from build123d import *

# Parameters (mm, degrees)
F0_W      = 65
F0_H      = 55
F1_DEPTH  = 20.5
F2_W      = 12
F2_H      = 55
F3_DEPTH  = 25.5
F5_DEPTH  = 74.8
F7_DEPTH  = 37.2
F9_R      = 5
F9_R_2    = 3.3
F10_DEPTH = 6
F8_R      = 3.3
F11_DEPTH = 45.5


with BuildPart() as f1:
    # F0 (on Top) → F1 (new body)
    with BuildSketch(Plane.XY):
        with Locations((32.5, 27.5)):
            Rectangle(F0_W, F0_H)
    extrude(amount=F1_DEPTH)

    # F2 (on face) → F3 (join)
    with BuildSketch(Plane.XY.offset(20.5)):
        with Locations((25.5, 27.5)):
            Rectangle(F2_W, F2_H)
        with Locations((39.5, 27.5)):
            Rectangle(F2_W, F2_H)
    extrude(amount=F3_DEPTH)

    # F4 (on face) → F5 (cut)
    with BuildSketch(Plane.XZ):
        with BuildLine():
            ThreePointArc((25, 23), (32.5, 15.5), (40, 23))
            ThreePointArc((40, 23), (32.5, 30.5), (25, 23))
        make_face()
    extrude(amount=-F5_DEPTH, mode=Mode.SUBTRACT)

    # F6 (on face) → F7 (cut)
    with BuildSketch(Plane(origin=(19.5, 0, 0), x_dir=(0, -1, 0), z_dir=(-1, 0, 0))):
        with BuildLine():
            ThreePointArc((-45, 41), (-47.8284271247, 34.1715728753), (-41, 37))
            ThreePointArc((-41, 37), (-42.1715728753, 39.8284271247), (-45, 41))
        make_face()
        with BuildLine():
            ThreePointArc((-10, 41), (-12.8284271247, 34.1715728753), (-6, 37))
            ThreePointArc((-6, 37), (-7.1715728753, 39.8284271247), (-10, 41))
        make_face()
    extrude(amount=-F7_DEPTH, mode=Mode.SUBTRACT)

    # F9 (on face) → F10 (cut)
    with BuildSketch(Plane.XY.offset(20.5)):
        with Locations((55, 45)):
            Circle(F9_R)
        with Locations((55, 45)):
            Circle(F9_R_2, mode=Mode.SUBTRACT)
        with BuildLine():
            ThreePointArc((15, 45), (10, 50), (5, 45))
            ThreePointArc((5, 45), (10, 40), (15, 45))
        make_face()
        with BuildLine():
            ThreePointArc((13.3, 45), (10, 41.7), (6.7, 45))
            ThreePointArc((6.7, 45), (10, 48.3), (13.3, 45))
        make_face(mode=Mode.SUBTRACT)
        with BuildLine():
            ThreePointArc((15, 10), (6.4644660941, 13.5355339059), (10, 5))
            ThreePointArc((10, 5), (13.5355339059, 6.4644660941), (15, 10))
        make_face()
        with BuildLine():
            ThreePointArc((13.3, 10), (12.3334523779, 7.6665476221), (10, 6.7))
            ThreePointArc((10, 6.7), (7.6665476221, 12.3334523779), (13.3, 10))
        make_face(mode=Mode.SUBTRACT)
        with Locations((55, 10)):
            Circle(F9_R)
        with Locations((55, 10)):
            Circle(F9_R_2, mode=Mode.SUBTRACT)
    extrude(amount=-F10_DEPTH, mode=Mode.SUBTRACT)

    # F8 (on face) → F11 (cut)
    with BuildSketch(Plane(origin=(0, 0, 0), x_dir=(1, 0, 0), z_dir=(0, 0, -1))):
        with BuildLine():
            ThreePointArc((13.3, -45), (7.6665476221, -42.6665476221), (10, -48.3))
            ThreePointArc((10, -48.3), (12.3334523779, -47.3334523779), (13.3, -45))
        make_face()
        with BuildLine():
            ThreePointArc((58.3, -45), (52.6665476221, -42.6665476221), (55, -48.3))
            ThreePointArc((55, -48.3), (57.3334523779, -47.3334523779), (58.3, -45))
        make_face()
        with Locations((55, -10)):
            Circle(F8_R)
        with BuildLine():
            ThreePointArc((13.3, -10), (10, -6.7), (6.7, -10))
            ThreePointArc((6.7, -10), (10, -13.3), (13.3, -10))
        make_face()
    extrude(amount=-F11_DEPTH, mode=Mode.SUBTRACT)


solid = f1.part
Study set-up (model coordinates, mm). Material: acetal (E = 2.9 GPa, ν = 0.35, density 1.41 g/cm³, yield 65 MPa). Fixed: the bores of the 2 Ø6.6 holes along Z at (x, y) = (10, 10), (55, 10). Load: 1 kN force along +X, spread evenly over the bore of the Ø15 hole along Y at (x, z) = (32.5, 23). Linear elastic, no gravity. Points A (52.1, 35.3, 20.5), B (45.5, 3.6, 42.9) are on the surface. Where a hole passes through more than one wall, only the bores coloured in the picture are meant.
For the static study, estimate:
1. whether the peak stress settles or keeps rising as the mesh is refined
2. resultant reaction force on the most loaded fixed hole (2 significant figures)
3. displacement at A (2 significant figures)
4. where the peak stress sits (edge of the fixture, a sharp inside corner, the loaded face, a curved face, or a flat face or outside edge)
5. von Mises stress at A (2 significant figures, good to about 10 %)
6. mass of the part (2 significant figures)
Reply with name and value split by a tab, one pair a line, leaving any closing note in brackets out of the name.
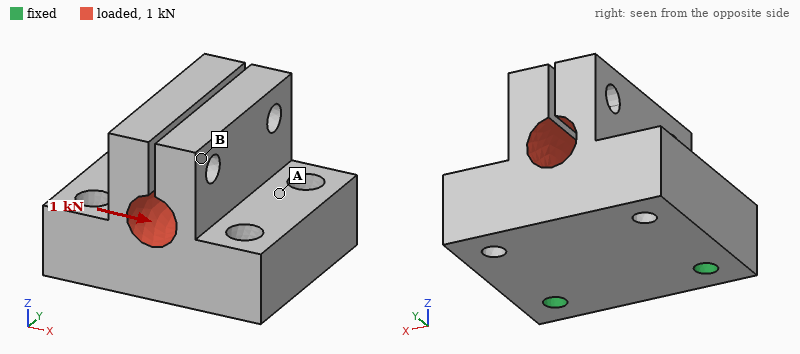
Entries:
whether the peak stress settles or keeps rising as the mesh is refined	keeps rising
resultant reaction force on the most loaded fixed hole	680 N
displacement at A	0.035 mm
where the peak stress sits	edge of the fixture
von Mises stress at A	1.4 MPa
mass of the part	130 g
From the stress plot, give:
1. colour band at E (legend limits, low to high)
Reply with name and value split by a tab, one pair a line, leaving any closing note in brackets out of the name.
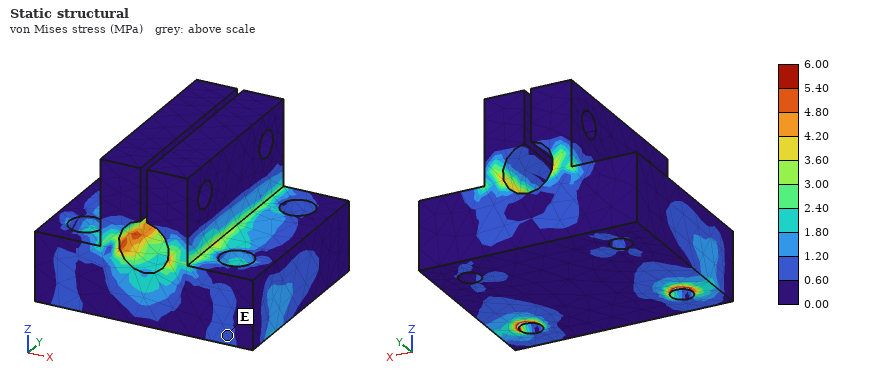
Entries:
colour band at E	0.60 to 1.20 MPa
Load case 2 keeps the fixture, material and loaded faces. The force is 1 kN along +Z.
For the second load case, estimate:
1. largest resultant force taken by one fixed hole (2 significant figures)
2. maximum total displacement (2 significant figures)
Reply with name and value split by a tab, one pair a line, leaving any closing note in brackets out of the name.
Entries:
largest resultant force taken by one fixed hole	510 N
maximum total displacement	0.31 mm
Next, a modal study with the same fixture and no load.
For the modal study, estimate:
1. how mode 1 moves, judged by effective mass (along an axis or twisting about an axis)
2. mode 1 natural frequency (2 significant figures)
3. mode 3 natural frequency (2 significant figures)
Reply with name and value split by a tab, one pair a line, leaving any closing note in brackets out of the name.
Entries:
how mode 1 moves, judged by effective mass	along Z
mode 1 natural frequency	1100 Hz
mode 3 natural frequency	1200 Hz
